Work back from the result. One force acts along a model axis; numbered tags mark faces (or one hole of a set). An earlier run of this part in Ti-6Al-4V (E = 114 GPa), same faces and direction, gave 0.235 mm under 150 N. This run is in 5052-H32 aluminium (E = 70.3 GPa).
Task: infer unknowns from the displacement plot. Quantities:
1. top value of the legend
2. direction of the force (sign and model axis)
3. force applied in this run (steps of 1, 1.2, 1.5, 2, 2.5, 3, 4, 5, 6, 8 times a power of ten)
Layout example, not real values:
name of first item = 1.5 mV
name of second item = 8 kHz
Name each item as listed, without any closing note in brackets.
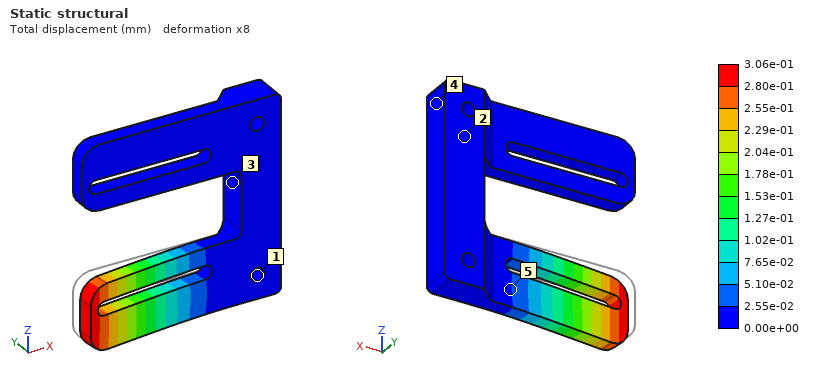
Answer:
top value of the legend = 3.06e-01 mm
direction of the force = -Y
force applied in this run = 120 N
